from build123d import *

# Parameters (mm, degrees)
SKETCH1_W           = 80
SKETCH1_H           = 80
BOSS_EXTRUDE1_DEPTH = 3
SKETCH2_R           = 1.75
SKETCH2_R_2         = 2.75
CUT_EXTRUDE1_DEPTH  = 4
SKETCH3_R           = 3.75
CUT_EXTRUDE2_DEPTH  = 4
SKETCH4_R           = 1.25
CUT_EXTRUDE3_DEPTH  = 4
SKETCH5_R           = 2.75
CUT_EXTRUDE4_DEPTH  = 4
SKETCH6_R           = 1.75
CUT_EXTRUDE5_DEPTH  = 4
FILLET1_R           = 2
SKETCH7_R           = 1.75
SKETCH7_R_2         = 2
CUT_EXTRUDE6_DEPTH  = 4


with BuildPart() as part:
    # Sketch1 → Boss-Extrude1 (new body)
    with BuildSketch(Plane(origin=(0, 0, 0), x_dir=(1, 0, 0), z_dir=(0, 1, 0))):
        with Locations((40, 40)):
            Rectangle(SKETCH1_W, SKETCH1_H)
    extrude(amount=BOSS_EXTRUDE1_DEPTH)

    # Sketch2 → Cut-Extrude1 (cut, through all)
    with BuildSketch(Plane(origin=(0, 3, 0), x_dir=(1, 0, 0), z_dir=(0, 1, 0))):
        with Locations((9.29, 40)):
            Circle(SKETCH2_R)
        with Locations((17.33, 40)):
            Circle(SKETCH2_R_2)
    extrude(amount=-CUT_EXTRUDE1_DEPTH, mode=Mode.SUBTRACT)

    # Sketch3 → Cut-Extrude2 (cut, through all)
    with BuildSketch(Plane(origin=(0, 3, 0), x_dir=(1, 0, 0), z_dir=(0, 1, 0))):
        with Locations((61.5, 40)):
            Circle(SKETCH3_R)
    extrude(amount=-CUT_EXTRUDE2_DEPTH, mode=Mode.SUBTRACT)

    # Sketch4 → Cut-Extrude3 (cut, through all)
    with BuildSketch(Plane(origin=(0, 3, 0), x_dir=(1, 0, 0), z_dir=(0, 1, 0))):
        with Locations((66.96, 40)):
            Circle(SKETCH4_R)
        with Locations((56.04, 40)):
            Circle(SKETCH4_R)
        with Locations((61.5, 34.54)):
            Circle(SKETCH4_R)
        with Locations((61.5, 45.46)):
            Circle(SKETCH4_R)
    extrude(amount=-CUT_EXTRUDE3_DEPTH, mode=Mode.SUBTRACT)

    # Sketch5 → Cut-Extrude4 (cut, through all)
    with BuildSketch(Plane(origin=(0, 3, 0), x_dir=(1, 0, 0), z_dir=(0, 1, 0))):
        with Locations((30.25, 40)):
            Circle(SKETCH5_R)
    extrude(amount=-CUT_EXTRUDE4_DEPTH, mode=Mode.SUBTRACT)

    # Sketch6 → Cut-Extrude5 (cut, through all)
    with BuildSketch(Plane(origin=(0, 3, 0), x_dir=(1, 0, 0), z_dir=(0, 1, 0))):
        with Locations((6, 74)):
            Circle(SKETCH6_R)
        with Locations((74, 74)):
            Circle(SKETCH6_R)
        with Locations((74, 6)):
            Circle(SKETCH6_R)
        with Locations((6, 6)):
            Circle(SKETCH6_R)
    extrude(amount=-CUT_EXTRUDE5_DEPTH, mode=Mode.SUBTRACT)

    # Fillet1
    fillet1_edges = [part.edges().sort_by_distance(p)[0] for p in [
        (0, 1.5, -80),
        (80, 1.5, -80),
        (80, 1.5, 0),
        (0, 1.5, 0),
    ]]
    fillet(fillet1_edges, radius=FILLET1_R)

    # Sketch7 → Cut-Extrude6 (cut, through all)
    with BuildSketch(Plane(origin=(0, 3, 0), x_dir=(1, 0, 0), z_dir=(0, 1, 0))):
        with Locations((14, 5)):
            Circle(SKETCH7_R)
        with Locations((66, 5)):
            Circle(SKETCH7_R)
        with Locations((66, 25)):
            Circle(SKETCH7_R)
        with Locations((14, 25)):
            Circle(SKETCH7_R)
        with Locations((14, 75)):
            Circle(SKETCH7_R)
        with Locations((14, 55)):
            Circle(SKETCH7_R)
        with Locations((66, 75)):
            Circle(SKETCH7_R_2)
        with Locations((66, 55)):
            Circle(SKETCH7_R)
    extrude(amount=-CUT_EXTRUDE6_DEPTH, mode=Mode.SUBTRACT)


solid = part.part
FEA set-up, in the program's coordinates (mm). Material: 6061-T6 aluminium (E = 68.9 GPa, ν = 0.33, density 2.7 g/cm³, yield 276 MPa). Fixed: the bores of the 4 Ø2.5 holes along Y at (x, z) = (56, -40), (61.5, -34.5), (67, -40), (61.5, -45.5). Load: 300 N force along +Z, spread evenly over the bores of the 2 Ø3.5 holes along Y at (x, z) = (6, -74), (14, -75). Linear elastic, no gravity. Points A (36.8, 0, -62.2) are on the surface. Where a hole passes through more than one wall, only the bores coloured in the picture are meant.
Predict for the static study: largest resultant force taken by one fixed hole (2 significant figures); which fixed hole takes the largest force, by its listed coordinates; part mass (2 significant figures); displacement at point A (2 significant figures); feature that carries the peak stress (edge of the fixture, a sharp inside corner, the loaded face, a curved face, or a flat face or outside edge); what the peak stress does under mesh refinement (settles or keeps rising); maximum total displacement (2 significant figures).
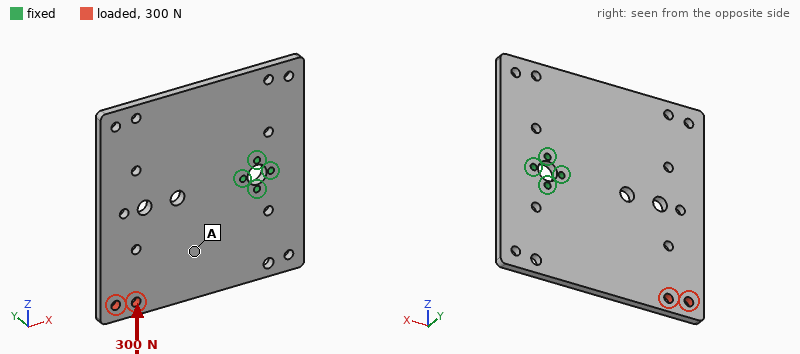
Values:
750 N
(56, -40)
50 g
17 µm
edge of the fixture
keeps rising
40 µm
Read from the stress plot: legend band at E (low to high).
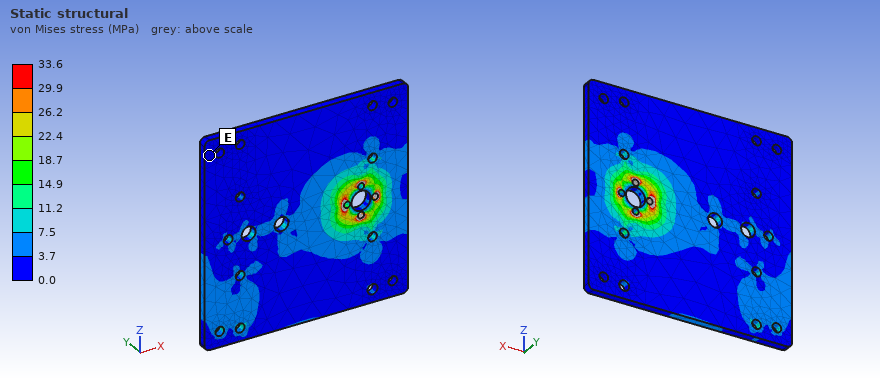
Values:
0.0 to 3.7 MPa
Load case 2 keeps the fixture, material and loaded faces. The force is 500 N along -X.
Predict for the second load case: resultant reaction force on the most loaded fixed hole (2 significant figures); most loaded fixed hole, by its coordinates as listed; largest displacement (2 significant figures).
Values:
880 N
(61.5, -45.5)
47 µm
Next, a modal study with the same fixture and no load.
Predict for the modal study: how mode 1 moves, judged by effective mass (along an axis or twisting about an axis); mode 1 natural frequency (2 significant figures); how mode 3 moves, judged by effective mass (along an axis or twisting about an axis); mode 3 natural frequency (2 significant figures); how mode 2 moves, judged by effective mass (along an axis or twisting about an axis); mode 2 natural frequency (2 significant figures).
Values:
along Y
640 Hz
along Y
1900 Hz
twisting about X
900 Hz
